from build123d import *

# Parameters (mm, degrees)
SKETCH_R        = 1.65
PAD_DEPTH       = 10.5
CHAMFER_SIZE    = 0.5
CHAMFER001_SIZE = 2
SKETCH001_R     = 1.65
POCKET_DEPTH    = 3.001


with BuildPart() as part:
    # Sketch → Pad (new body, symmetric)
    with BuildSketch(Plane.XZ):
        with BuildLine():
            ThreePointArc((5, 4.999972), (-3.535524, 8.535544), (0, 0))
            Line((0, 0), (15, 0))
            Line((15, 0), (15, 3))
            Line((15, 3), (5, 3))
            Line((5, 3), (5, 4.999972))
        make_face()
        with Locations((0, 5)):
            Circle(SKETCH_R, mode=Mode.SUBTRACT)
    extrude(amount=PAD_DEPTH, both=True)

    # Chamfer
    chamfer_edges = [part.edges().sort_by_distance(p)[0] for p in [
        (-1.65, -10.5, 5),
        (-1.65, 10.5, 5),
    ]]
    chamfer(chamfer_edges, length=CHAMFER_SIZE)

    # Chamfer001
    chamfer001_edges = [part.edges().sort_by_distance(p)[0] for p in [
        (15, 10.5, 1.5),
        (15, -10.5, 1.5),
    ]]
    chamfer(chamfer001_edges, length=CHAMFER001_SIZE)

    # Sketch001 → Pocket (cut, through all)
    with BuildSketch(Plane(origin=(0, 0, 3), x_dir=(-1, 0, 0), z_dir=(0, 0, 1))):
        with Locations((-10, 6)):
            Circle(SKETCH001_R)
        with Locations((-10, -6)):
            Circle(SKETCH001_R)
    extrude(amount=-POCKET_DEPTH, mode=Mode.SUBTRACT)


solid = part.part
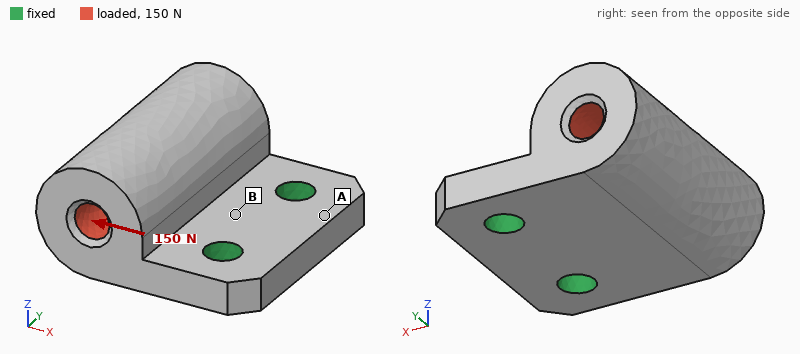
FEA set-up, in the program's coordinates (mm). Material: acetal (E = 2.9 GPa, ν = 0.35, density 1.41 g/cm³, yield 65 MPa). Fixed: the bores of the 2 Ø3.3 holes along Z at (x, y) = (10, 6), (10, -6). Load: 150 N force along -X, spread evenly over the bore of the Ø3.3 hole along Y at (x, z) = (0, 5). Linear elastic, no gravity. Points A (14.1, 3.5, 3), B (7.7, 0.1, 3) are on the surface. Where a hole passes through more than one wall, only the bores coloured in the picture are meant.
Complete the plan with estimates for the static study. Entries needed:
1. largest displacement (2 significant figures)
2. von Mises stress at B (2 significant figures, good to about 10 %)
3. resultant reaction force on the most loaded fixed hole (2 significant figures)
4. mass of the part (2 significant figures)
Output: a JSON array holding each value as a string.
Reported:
["0.26 mm", "12 MPa", "76 N", "3.0 g"]
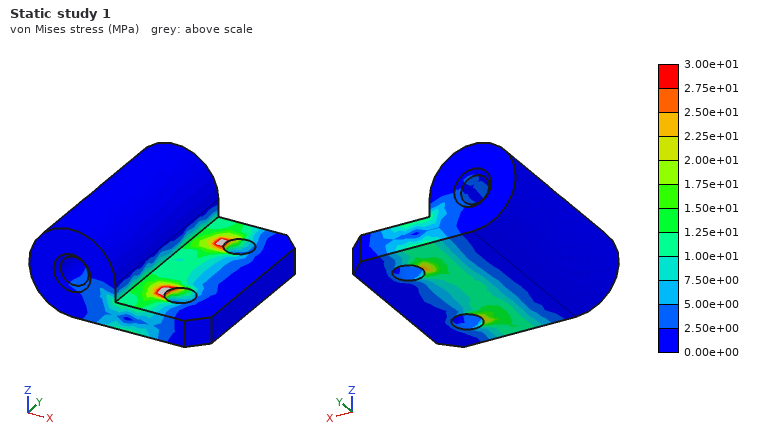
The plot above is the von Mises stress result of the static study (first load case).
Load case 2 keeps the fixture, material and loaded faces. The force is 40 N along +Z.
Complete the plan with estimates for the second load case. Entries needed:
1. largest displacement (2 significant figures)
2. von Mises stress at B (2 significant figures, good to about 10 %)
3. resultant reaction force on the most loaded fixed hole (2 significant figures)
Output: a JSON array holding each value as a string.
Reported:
["0.14 mm", "5.6 MPa", "20 N"]
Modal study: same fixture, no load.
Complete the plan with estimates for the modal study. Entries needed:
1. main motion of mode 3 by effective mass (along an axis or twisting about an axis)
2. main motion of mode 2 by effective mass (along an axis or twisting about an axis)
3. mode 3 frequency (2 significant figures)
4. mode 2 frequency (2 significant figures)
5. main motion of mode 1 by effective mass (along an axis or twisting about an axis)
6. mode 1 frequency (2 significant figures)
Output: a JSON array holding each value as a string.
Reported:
["along Y", "along Y", "7700 Hz", "5400 Hz", "along Z", "2000 Hz"]
